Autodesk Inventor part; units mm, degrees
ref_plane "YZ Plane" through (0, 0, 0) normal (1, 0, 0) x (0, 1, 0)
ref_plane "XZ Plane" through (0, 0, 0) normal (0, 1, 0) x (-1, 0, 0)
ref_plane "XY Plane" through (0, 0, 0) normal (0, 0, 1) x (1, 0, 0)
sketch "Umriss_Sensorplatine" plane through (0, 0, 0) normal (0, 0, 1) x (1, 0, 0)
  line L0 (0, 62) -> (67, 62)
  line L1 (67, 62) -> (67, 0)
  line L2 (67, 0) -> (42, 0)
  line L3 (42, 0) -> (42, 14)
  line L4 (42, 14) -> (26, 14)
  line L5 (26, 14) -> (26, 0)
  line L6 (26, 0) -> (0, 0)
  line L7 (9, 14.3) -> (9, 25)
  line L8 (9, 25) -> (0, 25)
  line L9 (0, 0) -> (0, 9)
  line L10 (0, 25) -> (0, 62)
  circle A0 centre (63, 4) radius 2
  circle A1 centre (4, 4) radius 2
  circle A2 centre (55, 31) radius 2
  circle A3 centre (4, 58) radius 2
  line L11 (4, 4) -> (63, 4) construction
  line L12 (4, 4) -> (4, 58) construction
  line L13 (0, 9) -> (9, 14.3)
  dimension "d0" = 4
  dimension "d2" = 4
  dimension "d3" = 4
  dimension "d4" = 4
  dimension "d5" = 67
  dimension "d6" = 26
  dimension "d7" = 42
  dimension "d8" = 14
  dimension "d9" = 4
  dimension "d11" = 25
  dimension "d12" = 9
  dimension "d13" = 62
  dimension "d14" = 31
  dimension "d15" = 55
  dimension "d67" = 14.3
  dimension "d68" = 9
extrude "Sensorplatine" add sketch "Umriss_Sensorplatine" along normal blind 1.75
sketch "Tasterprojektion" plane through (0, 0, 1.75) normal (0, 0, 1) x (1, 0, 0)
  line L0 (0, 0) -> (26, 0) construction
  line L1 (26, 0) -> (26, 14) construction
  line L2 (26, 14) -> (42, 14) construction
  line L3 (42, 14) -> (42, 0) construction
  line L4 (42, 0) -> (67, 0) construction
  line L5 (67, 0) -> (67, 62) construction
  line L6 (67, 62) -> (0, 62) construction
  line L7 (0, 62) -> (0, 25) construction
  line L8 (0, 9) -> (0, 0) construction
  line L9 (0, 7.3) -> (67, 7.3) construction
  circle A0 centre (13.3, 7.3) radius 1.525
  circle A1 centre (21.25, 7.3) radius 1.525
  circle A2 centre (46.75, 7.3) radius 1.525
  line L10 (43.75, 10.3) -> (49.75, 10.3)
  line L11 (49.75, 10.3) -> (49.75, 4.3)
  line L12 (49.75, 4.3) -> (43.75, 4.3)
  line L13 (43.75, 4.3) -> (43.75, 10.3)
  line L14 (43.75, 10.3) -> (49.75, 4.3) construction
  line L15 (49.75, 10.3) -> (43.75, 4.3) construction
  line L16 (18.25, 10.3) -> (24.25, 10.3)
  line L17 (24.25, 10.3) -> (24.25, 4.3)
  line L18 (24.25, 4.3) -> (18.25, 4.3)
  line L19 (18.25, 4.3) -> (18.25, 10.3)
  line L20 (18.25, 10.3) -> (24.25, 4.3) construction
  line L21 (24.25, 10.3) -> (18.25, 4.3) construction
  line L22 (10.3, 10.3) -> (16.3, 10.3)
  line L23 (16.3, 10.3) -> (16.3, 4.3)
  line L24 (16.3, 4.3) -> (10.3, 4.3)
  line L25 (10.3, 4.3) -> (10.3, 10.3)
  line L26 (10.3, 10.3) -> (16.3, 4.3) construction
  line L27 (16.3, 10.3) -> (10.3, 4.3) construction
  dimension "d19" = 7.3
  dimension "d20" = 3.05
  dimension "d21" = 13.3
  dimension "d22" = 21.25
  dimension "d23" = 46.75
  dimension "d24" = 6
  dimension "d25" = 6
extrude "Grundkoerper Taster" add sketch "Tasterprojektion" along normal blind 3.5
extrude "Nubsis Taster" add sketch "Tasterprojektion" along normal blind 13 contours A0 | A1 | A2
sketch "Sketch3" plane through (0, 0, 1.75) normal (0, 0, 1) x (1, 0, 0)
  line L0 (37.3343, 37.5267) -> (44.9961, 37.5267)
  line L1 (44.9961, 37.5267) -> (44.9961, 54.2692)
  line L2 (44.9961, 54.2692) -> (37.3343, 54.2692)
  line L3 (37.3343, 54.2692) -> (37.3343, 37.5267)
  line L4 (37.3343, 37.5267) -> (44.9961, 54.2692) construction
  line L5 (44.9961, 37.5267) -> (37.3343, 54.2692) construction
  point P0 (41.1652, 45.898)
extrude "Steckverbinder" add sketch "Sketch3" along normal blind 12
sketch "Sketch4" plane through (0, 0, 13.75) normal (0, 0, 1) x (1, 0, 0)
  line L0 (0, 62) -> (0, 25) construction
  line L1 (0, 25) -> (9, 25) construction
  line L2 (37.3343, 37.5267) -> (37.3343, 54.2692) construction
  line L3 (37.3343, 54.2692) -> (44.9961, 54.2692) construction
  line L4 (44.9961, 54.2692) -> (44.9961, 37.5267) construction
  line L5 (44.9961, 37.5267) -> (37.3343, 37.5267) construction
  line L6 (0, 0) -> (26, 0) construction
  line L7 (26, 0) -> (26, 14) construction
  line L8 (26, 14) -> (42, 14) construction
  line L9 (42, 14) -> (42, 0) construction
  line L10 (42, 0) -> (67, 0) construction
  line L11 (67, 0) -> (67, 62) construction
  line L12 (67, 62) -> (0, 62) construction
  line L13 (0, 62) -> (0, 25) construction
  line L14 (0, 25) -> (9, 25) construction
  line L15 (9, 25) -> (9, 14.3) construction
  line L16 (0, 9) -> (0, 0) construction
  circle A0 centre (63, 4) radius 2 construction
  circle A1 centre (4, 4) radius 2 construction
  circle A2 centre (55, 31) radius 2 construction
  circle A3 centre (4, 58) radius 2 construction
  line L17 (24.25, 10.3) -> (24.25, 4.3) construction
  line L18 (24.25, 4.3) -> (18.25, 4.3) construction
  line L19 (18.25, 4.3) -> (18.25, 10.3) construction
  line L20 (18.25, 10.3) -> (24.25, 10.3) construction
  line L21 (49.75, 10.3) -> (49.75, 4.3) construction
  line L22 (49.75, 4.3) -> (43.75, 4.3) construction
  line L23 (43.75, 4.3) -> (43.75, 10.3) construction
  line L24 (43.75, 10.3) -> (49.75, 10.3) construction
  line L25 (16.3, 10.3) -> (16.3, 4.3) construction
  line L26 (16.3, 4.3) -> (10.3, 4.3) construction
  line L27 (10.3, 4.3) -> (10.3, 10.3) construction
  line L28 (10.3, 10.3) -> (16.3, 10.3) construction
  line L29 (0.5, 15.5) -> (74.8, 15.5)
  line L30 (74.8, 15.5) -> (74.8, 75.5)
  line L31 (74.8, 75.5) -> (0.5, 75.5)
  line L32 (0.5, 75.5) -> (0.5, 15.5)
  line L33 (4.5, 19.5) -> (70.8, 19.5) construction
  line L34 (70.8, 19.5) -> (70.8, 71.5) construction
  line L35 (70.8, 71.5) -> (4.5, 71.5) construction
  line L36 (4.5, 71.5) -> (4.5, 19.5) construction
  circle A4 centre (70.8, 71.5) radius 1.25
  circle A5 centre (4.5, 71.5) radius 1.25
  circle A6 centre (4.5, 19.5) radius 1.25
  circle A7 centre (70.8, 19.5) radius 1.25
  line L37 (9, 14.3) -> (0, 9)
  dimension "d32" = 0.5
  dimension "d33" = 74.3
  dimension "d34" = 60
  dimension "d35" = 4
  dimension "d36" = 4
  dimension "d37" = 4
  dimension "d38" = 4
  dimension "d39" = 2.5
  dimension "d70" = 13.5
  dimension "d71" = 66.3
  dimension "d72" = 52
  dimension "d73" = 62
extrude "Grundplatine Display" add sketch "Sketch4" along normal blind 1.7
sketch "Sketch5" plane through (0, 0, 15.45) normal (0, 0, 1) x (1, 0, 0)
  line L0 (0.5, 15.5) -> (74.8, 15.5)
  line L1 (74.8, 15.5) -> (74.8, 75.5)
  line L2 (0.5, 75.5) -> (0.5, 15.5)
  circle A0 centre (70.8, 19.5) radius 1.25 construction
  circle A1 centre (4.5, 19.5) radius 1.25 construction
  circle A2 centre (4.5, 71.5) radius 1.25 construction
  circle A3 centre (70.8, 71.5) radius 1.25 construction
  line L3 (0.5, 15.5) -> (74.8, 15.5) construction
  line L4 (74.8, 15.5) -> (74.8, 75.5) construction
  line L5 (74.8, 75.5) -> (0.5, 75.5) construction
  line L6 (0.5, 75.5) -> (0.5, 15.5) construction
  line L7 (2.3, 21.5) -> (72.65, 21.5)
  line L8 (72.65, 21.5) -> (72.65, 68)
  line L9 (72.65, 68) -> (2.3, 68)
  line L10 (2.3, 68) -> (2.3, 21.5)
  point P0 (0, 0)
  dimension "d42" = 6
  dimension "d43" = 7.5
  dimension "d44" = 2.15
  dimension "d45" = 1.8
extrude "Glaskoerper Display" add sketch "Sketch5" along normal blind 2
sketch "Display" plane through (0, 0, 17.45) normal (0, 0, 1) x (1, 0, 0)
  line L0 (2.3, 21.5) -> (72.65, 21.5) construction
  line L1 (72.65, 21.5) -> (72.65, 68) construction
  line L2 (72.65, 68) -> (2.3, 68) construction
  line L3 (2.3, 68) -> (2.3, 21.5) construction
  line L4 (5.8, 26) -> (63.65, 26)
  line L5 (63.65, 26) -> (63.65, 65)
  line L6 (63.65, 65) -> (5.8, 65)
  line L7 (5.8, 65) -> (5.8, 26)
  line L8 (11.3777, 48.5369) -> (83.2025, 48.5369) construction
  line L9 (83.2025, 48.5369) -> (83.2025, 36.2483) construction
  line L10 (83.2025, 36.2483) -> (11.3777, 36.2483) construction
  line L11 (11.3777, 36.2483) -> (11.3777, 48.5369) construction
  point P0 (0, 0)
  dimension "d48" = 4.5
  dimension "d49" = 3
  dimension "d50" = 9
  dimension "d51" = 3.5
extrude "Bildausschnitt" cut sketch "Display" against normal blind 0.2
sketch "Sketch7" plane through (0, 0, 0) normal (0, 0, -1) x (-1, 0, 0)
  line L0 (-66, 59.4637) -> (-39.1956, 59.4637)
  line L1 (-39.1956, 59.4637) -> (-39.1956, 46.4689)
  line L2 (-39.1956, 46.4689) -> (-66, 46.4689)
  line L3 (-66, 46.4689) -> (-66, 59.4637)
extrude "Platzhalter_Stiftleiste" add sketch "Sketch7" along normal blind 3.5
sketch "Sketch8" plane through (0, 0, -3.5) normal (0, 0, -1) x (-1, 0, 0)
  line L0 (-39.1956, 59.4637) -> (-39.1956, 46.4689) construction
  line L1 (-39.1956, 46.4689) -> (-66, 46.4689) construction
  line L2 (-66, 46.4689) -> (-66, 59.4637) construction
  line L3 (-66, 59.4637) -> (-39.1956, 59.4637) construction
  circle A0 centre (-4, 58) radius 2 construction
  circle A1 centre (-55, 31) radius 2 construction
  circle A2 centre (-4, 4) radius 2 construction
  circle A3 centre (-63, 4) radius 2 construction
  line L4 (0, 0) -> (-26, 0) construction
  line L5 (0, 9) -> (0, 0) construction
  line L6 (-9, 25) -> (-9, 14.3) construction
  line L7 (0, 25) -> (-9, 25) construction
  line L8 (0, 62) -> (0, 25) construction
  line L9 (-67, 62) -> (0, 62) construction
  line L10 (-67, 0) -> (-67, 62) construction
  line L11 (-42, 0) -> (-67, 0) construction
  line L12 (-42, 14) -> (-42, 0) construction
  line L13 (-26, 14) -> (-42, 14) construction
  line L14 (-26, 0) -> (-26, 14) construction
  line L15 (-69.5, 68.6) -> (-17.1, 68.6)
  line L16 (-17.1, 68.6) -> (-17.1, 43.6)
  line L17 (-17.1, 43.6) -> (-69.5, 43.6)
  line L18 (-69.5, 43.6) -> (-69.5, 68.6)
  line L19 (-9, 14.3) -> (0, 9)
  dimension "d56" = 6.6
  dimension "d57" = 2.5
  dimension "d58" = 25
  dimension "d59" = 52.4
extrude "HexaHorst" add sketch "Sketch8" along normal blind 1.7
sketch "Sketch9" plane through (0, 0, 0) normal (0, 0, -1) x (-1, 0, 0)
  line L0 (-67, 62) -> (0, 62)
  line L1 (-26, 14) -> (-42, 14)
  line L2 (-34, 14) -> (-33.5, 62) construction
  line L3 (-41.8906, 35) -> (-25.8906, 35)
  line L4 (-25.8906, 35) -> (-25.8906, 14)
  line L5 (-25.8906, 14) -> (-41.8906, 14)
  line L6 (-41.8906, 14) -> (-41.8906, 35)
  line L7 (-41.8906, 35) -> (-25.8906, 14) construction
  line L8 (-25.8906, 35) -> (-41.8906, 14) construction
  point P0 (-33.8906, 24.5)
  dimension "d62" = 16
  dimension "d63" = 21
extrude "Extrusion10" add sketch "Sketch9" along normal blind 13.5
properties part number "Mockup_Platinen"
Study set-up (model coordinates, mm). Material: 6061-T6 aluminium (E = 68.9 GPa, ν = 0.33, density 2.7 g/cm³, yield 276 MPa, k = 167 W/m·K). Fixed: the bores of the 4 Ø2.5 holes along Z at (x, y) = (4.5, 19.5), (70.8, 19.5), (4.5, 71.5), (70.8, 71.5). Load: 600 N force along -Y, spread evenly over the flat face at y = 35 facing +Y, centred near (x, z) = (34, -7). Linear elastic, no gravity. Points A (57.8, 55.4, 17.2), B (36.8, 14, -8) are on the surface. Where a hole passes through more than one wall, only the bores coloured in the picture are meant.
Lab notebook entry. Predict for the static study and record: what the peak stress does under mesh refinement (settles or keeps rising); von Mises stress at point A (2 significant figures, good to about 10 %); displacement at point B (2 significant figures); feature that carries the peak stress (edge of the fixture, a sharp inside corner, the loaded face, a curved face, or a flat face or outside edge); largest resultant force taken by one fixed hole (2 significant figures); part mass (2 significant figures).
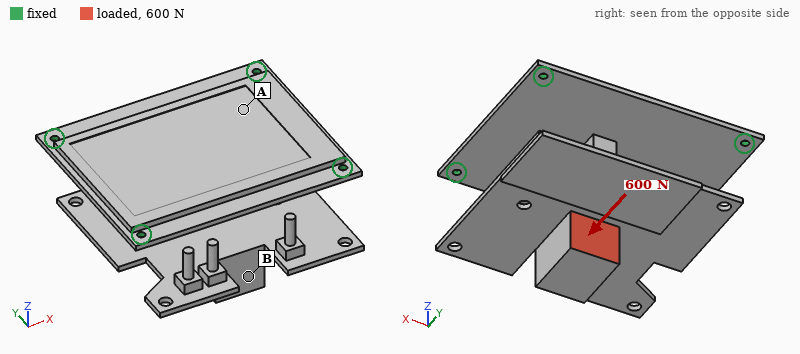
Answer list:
keeps rising
37 MPa
0.84 mm
edge of the fixture
210 N
82 g
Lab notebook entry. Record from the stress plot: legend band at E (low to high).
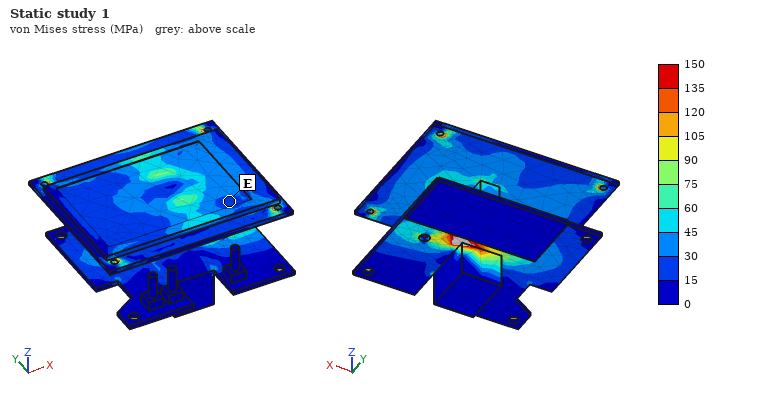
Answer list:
15 to 30 MPa
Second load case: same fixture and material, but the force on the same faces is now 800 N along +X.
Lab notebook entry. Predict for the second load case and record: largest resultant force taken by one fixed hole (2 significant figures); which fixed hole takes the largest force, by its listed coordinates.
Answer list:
370 N
(70.8, 19.5)
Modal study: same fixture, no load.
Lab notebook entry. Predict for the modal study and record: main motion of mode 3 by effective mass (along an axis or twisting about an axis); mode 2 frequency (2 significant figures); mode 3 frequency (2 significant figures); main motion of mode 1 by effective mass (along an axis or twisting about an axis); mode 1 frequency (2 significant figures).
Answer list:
along Z
960 Hz
1400 Hz
along Z
600 Hz
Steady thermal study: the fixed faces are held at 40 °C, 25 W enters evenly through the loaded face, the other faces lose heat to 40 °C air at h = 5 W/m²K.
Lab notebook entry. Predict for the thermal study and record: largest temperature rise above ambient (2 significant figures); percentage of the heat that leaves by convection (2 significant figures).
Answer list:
69 K
14 %
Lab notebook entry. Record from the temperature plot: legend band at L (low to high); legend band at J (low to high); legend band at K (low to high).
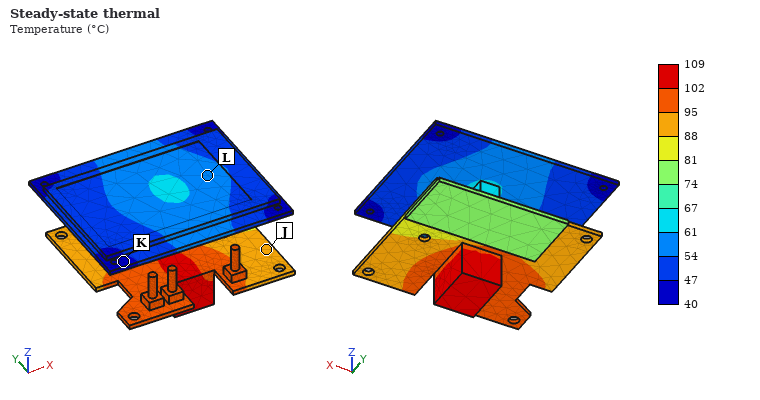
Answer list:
54 to 61 °C
88 to 95 °C
40 to 47 °C
